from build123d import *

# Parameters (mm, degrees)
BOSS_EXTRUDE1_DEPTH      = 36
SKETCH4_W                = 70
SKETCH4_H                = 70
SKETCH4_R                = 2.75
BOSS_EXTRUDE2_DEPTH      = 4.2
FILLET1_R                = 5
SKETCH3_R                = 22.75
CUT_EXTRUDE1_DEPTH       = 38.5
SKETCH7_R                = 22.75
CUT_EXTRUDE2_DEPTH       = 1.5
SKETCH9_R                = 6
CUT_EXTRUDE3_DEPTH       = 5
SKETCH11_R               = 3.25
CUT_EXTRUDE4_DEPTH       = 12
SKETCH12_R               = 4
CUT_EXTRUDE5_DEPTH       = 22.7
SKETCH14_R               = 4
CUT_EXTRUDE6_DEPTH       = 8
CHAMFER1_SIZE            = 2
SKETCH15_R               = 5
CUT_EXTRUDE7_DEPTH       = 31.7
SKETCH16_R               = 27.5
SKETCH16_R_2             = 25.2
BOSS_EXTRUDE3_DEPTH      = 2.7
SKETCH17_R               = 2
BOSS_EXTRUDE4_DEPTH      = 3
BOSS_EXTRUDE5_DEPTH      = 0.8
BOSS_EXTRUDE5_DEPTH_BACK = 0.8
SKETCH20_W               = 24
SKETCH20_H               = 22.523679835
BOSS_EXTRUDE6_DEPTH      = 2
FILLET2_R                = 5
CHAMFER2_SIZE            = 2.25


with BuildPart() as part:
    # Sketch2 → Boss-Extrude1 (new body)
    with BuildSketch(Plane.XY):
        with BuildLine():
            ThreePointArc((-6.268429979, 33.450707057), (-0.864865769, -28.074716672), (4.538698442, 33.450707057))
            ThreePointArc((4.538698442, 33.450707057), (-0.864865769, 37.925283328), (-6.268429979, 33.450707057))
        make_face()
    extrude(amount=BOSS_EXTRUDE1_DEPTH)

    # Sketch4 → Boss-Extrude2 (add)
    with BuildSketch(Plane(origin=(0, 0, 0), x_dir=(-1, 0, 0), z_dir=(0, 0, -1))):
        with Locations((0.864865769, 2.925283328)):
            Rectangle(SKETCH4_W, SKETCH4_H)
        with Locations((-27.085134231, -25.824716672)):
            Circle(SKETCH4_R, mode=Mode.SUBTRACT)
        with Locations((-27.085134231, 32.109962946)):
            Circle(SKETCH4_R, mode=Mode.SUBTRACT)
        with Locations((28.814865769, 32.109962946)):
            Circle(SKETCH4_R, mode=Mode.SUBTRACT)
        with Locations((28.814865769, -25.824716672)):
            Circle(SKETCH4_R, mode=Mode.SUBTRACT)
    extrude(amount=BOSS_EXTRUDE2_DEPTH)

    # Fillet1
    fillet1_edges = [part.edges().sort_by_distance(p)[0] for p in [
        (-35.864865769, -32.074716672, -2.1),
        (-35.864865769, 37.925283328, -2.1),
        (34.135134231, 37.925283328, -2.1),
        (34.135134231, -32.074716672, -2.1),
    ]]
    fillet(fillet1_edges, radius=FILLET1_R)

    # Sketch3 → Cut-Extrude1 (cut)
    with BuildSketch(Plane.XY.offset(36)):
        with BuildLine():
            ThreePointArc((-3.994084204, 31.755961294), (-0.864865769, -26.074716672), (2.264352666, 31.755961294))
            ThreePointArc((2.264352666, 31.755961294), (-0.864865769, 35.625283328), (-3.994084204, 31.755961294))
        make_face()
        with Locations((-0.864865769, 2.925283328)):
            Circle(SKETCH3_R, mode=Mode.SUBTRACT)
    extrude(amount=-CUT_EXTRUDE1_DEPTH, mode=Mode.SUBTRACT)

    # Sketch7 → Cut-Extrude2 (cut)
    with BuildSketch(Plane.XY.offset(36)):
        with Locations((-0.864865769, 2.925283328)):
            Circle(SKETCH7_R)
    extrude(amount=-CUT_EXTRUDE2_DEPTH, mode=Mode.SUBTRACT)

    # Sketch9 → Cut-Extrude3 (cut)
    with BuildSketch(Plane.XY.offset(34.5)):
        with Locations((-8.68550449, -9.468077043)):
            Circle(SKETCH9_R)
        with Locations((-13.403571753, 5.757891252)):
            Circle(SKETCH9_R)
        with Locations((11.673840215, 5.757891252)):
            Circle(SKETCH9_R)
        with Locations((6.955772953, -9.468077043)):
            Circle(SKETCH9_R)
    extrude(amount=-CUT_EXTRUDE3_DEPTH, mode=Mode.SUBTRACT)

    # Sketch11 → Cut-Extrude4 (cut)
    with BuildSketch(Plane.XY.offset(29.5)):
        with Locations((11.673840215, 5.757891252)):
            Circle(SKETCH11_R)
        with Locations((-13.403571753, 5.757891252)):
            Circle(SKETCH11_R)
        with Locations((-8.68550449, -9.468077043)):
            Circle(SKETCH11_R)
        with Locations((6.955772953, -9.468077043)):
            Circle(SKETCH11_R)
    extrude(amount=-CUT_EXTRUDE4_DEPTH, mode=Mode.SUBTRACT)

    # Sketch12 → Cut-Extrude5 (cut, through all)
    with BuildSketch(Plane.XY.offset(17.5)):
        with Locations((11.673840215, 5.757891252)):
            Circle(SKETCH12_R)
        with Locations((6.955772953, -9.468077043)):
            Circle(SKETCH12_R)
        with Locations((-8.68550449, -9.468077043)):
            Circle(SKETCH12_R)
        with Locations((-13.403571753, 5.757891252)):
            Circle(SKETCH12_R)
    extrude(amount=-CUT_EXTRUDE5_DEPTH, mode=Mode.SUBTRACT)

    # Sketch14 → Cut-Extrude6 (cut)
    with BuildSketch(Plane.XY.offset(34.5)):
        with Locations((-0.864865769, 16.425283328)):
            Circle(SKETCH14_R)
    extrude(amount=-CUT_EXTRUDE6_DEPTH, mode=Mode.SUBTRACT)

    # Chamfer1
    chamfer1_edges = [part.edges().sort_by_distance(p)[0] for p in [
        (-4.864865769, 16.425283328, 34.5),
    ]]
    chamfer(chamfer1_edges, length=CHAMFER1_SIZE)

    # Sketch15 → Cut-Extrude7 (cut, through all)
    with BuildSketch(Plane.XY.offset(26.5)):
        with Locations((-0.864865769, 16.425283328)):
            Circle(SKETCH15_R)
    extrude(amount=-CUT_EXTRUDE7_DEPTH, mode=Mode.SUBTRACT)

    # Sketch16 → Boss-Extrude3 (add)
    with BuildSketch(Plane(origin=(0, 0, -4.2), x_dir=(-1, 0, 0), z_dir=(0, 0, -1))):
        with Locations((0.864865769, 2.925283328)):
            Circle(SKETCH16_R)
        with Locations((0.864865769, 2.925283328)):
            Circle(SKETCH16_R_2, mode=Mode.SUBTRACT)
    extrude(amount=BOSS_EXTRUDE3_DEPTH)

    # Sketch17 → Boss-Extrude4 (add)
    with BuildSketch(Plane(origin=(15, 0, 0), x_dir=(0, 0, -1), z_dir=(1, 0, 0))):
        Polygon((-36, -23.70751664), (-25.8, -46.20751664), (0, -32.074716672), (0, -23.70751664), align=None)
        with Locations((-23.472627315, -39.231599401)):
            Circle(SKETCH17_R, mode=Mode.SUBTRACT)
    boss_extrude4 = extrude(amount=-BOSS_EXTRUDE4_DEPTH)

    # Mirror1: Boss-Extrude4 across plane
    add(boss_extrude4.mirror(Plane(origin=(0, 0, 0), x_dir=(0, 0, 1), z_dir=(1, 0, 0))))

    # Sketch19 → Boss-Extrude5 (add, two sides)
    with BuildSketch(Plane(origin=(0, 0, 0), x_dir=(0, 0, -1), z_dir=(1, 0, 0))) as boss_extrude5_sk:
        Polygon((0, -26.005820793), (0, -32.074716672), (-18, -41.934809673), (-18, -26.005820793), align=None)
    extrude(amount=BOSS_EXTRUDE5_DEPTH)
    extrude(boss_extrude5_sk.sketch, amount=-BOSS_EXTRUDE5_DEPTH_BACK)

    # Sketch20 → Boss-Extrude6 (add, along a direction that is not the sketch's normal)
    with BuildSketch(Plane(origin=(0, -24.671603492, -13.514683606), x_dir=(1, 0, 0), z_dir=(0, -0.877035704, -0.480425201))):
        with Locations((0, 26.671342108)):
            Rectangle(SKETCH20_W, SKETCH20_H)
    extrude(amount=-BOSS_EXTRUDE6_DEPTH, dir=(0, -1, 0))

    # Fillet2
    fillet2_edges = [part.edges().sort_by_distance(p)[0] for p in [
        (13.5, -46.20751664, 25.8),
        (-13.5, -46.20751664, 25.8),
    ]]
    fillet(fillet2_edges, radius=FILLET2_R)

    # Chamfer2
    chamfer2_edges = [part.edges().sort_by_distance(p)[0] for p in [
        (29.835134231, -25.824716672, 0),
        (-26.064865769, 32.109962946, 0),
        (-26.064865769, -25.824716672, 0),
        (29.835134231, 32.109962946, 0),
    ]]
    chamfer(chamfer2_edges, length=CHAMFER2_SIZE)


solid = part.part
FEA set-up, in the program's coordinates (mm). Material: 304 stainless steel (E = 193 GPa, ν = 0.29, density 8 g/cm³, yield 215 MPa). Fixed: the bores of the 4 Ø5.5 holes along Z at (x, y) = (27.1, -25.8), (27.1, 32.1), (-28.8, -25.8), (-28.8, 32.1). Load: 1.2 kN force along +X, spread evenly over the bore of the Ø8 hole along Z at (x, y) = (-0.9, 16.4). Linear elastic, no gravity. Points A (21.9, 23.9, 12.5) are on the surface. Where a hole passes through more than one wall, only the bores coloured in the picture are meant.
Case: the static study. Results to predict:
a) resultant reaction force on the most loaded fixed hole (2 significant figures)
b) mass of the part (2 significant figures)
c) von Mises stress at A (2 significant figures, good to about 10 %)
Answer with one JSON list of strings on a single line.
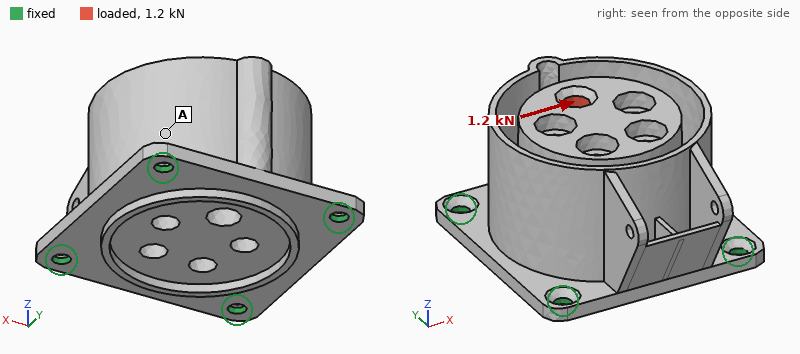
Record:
["610 N", "650 g", "7.5 MPa"]
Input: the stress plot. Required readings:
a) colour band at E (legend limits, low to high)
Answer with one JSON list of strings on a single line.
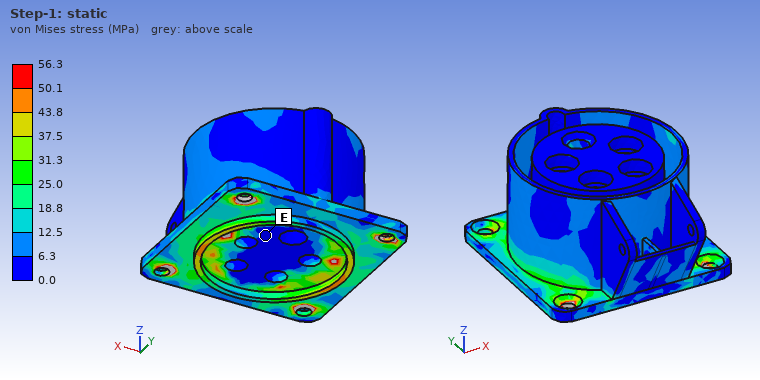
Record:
["0.0 to 6.3 MPa"]
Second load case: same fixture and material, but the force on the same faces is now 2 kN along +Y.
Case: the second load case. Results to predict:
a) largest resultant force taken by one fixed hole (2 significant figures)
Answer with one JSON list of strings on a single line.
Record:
["960 N"]
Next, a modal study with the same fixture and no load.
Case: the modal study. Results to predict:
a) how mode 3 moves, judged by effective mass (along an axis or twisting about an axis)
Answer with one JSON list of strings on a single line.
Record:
["along Z"]
